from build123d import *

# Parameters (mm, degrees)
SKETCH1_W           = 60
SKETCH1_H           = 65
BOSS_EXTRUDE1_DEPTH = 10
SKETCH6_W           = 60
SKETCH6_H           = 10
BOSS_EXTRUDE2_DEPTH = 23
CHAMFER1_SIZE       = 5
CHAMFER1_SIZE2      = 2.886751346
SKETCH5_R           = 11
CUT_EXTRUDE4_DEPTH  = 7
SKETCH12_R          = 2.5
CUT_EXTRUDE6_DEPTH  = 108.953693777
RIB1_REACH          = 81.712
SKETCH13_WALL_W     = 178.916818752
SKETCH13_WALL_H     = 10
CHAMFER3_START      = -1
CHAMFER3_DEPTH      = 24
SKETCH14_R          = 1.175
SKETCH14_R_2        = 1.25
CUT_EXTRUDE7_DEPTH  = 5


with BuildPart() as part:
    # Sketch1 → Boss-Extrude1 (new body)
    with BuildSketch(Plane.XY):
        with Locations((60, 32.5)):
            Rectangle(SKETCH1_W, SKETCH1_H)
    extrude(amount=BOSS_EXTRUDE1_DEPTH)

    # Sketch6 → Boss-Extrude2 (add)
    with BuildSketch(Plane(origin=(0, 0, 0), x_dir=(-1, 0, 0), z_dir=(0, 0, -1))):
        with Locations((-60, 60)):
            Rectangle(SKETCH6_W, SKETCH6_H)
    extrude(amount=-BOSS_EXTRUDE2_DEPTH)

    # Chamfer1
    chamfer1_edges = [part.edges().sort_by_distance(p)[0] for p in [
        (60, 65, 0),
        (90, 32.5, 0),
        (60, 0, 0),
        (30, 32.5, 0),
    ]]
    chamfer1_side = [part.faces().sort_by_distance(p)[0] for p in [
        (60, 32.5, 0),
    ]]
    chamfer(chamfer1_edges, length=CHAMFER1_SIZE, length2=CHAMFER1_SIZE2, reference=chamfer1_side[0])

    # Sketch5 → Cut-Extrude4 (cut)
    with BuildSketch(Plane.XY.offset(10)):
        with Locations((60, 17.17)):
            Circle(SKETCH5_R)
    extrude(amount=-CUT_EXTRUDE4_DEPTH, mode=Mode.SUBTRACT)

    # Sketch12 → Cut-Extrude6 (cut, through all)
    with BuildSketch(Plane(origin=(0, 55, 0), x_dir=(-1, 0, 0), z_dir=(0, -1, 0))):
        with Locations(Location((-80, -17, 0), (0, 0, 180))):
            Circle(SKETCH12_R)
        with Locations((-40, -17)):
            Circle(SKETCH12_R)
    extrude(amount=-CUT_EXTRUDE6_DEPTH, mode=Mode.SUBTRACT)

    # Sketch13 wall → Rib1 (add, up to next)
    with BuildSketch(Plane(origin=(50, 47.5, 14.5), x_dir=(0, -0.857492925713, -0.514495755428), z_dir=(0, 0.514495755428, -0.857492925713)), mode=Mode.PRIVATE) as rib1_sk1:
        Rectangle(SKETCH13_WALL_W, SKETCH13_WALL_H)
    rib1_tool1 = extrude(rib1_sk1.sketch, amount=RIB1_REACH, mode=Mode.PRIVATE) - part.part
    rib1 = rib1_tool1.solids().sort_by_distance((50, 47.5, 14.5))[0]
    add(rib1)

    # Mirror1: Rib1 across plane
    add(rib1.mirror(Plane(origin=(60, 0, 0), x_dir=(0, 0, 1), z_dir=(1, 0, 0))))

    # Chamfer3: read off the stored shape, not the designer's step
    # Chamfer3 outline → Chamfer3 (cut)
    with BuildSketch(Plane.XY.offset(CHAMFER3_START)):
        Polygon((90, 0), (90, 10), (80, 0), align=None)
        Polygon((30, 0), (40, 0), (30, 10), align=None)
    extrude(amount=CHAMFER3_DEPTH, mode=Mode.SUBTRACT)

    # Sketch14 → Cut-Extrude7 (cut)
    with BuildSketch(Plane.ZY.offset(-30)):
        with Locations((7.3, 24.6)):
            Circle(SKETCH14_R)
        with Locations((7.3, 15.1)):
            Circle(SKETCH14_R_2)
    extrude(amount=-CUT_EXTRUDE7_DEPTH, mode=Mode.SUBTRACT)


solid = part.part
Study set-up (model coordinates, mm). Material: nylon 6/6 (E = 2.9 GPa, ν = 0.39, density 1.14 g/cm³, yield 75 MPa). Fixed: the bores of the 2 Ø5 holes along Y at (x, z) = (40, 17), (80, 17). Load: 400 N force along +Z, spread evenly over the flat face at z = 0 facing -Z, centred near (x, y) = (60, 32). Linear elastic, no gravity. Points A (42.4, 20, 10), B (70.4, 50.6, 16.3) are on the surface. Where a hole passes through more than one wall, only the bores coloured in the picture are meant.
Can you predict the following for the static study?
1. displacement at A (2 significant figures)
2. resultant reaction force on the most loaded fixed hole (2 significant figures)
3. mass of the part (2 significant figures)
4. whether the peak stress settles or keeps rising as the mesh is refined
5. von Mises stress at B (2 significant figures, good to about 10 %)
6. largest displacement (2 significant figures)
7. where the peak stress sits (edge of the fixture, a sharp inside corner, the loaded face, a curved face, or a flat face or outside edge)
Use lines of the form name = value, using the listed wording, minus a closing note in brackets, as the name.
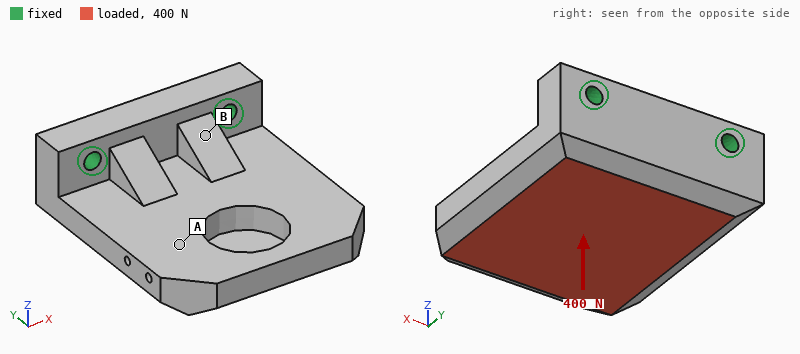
displacement at A = 0.54 mm
resultant reaction force on the most loaded fixed hole = 220 N
mass of the part = 48 g
whether the peak stress settles or keeps rising as the mesh is refined = keeps rising
von Mises stress at B = 7.4 MPa
largest displacement = 0.92 mm
where the peak stress sits = edge of the fixture
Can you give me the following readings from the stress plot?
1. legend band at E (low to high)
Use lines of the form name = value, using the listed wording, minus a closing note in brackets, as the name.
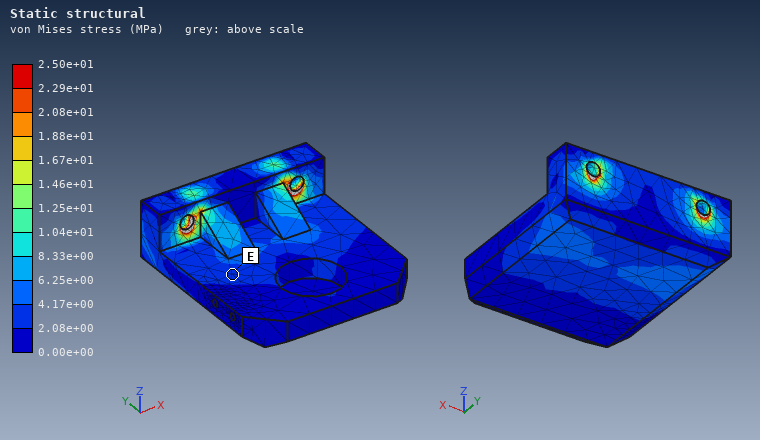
legend band at E = 2.08e+00 to 4.17e+00 MPa
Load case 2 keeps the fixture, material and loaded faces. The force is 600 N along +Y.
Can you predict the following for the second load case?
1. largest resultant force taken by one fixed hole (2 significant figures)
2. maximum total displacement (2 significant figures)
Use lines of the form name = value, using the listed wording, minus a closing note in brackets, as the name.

largest resultant force taken by one fixed hole = 300 N
maximum total displacement = 0.60 mm
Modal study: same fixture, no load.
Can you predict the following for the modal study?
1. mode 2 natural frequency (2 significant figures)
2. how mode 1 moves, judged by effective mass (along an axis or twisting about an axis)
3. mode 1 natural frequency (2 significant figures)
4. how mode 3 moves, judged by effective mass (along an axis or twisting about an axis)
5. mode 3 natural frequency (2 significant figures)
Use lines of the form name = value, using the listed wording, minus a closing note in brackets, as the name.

mode 2 natural frequency = 1500 Hz
how mode 1 moves, judged by effective mass = along Z
mode 1 natural frequency = 690 Hz
how mode 3 moves, judged by effective mass = along X
mode 3 natural frequency = 2100 Hz
